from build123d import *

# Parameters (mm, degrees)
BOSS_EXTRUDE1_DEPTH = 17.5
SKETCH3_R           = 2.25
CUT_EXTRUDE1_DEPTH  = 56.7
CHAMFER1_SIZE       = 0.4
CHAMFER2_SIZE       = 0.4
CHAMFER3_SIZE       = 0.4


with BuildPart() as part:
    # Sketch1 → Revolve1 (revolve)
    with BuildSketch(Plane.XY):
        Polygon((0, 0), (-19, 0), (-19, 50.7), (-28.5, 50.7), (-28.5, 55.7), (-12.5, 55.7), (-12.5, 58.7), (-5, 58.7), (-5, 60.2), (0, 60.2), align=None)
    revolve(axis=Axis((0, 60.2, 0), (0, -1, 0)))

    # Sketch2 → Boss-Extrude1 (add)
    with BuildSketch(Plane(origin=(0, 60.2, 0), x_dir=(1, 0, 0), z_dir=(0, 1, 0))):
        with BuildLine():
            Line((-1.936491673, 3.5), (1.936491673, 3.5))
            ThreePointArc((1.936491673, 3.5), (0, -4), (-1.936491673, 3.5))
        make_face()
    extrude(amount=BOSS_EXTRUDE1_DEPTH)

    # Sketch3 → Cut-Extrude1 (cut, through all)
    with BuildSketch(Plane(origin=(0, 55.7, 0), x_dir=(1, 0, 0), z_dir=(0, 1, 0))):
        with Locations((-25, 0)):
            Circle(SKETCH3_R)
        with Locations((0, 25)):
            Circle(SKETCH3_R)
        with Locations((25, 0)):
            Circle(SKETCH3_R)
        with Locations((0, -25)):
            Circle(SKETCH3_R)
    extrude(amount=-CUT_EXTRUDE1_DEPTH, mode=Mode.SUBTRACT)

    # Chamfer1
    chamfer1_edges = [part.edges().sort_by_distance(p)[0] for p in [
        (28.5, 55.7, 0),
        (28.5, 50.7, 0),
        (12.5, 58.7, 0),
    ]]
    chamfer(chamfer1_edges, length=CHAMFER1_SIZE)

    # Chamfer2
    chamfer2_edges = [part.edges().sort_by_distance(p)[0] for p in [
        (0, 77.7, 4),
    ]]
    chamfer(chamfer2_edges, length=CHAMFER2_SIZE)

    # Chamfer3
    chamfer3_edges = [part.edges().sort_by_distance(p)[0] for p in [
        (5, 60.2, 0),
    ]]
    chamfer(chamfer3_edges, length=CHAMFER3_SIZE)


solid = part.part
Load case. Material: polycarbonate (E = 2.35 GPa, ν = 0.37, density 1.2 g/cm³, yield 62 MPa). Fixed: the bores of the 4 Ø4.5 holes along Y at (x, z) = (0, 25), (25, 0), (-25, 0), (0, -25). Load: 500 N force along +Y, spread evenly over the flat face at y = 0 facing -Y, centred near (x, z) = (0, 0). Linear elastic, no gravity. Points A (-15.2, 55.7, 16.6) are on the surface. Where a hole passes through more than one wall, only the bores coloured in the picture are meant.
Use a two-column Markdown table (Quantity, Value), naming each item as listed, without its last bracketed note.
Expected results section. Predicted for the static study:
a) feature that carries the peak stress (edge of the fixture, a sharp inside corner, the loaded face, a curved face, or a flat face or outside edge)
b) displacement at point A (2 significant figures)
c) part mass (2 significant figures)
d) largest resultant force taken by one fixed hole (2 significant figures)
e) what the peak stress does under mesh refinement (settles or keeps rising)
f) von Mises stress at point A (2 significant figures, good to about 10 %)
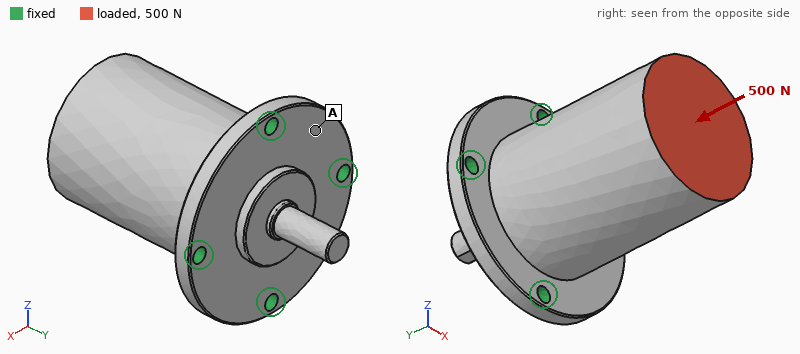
| Quantity | Value |
|---|---|
| feature that carries the peak stress | edge of the fixture |
| displacement at point A | 27 µm |
| part mass | 87 g |
| largest resultant force taken by one fixed hole | 130 N |
| what the peak stress does under mesh refinement | keeps rising |
| von Mises stress at point A | 1.4 MPa |
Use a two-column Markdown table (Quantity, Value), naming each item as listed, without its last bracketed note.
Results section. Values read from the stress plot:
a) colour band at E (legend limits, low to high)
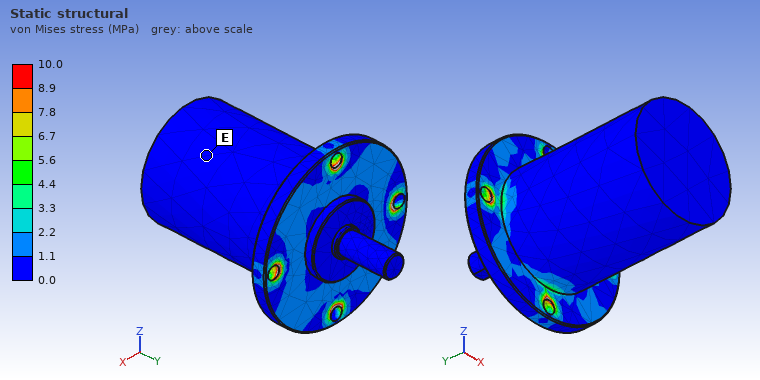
| Quantity | Value |
|---|---|
| colour band at E | 0.0 to 1.1 MPa |
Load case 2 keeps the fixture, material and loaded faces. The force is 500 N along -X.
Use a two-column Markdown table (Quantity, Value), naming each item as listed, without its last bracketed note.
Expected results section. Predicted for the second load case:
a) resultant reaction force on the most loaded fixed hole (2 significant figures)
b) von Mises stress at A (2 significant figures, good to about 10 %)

| Quantity | Value |
|---|---|
| resultant reaction force on the most loaded fixed hole | 620 N |
| von Mises stress at A | 4.5 MPa |
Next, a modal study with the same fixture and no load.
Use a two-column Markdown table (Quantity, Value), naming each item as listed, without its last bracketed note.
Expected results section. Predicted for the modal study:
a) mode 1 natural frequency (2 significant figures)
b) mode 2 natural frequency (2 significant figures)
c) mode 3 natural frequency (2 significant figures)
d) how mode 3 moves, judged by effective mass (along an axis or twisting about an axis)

| Quantity | Value |
|---|---|
| mode 1 natural frequency | 1100 Hz |
| mode 2 natural frequency | 1100 Hz |
| mode 3 natural frequency | 2200 Hz |
| how mode 3 moves, judged by effective mass | along Y |
